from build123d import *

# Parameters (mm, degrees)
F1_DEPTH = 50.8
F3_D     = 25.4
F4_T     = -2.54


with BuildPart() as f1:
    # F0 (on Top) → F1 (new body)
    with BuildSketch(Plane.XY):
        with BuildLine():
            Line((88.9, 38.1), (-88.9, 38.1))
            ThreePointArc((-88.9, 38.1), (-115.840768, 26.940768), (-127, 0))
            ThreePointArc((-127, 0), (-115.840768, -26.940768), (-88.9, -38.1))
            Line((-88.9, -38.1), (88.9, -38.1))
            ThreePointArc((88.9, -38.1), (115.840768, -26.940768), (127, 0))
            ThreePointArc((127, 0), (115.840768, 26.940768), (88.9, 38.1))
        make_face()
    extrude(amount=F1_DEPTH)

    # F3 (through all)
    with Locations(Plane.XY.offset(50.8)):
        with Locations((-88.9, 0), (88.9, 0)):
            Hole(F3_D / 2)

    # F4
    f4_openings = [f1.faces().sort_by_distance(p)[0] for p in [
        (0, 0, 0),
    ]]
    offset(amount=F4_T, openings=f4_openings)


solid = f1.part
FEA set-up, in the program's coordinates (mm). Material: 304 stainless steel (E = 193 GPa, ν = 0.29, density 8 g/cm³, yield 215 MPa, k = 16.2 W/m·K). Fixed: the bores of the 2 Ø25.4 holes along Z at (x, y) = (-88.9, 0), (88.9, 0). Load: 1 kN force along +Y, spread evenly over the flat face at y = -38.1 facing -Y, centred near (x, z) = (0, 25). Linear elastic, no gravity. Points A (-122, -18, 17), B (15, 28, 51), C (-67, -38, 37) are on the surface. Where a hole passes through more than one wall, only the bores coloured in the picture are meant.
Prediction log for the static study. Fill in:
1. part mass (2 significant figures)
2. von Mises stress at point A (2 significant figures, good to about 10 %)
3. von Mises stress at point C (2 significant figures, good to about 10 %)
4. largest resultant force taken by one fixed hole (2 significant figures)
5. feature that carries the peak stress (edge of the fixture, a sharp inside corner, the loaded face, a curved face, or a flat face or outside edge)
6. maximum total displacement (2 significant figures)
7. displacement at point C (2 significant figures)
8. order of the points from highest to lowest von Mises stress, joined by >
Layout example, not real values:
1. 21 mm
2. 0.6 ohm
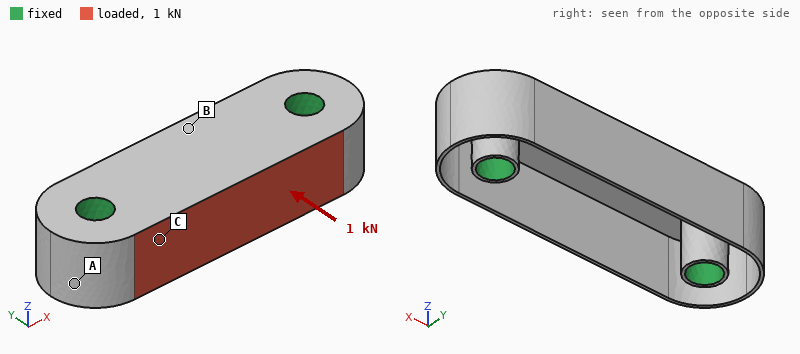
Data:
1. 1.1 kg
2. 26 MPa
3. 43 MPa
4. 500 N
5. a flat face or outside edge
6. 0.58 mm
7. 0.11 mm
8. C > A > B
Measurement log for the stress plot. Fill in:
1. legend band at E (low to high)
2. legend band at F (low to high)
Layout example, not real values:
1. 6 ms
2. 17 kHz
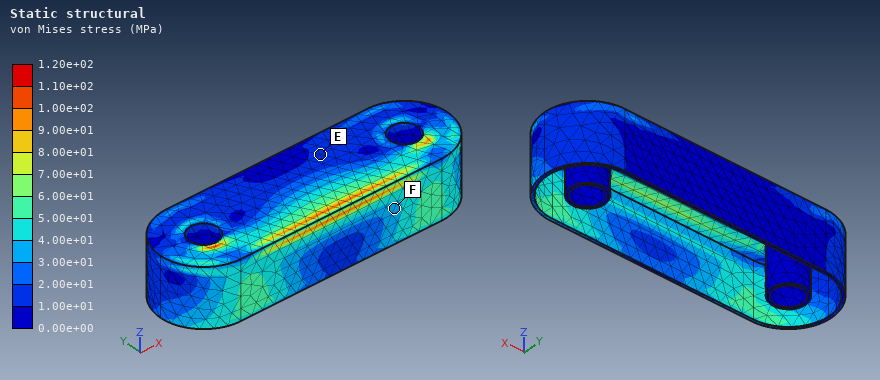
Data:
1. 1.00e+01 to 2.00e+01 MPa
2. 3.00e+01 to 4.00e+01 MPa
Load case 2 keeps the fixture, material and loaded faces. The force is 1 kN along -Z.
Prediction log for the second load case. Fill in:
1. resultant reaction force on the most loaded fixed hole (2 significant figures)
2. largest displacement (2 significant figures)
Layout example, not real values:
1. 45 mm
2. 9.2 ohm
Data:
1. 590 N
2. 0.20 mm
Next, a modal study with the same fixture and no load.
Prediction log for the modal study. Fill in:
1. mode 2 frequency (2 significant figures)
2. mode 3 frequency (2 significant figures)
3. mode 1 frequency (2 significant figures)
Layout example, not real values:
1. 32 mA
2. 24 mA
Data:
1. 610 Hz
2. 740 Hz
3. 600 Hz
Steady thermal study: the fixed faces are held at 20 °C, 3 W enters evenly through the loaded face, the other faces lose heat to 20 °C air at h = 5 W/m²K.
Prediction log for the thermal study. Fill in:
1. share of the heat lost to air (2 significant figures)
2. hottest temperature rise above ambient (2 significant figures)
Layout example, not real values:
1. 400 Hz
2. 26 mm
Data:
1. 54 %
2. 16 K
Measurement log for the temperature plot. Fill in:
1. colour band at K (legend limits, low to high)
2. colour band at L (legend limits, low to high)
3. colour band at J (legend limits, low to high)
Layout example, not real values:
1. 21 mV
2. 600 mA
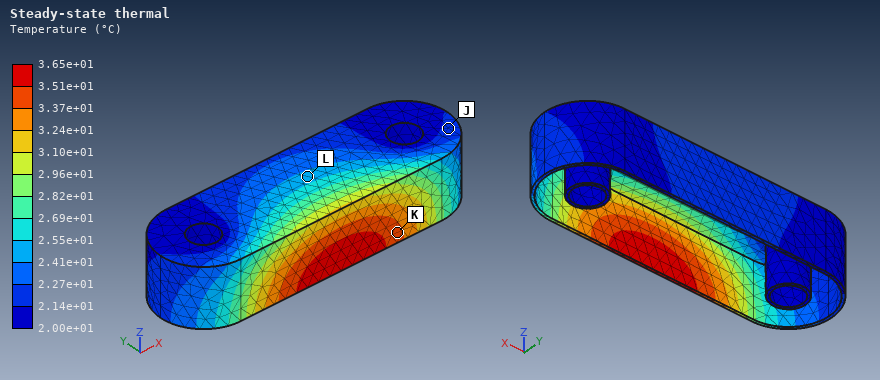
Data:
1. 3.37e+01 to 3.51e+01 °C
2. 2.41e+01 to 2.55e+01 °C
3. 2.14e+01 to 2.27e+01 °C
